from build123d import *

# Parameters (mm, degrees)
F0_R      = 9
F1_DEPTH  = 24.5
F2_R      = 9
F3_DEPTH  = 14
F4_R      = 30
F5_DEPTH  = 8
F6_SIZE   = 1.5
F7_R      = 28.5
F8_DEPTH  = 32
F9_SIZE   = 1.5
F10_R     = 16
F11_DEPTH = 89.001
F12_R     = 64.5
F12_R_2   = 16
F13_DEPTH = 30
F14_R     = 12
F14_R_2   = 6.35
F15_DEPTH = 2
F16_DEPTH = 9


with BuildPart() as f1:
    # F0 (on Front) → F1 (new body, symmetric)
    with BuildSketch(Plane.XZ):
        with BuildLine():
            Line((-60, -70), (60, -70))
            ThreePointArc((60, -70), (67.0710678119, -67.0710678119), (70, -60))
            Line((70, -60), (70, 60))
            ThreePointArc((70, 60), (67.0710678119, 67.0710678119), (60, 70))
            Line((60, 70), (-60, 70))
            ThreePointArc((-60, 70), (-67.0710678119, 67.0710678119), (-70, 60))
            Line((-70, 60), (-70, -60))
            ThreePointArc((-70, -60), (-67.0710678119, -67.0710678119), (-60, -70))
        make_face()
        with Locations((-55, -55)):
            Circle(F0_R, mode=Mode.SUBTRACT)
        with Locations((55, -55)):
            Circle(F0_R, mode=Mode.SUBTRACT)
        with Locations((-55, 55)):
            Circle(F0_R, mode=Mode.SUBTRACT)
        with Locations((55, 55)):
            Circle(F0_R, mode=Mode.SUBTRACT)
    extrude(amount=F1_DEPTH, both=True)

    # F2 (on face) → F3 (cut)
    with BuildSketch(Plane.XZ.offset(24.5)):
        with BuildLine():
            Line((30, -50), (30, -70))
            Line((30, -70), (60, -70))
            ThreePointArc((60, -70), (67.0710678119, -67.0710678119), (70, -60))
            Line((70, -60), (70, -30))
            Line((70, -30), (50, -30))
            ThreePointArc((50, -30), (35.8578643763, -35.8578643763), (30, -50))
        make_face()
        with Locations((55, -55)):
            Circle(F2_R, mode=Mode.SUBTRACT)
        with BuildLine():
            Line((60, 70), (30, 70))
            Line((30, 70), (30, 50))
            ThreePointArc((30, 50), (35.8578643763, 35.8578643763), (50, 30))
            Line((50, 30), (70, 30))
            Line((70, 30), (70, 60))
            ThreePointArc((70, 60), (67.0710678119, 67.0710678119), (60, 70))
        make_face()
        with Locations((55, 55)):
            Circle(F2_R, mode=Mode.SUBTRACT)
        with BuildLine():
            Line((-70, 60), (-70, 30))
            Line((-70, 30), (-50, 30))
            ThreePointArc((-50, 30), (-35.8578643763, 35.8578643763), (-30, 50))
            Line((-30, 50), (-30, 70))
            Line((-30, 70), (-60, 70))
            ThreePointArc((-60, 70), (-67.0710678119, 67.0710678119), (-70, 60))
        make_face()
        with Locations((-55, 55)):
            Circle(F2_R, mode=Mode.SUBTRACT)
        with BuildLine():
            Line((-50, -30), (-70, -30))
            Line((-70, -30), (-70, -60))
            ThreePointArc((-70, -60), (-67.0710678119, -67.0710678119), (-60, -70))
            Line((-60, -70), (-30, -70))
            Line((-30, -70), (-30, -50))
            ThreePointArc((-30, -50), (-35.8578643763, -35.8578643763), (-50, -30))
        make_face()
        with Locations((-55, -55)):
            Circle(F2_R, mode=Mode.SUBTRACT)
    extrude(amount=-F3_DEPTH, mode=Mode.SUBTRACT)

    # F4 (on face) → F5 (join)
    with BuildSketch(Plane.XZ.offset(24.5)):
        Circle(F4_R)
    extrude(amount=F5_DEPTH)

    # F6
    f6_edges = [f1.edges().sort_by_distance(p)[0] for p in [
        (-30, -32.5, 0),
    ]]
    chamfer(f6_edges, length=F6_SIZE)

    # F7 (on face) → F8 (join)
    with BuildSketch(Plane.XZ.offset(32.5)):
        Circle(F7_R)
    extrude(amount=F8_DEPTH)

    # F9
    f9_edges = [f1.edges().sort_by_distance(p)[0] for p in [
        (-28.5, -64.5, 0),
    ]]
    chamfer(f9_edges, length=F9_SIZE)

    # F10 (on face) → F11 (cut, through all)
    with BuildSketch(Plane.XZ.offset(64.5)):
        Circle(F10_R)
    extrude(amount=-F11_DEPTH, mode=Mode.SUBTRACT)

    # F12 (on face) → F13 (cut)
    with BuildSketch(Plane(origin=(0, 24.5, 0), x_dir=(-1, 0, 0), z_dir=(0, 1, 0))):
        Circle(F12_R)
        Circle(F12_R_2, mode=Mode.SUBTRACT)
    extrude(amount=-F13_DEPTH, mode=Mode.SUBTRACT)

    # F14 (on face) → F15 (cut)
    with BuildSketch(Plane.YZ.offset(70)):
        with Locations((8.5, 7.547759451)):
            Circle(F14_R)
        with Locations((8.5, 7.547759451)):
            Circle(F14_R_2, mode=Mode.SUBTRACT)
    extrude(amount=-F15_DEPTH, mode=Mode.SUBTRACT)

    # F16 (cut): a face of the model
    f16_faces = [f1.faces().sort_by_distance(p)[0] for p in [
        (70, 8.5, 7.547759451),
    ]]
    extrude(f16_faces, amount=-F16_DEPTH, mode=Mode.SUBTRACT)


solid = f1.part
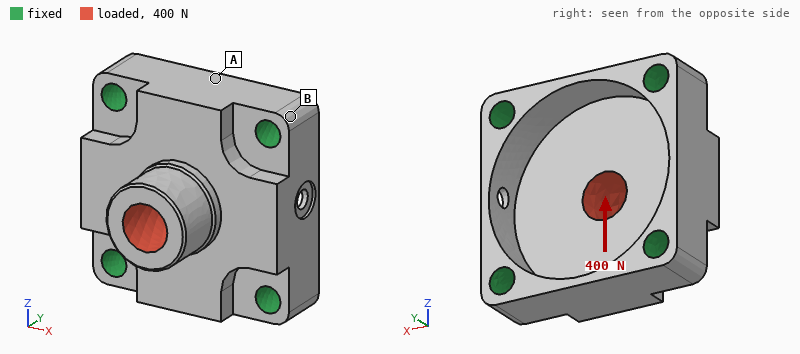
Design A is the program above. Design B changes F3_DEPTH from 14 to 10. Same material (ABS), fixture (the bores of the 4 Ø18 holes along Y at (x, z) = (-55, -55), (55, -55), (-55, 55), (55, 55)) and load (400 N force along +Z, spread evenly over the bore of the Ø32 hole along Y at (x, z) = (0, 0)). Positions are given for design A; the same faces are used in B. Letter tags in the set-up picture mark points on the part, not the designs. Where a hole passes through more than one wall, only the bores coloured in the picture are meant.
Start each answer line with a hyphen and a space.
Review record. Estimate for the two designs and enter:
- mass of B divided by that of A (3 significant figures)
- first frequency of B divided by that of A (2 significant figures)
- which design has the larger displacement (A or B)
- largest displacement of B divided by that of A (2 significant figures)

- 1.04
- 1.1
- A
- 0.91
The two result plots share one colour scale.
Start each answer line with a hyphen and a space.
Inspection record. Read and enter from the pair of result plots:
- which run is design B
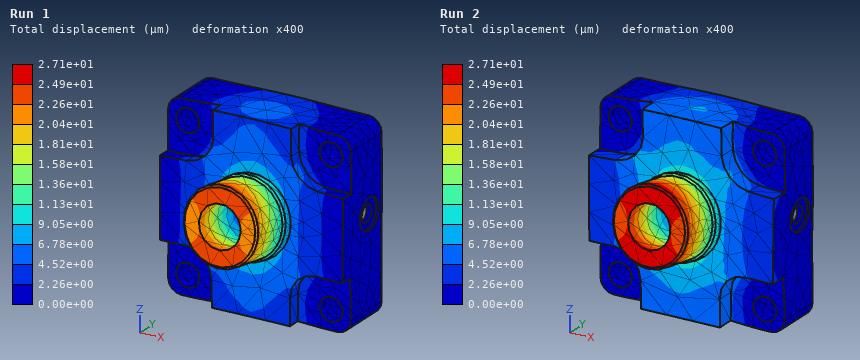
- Run 1
